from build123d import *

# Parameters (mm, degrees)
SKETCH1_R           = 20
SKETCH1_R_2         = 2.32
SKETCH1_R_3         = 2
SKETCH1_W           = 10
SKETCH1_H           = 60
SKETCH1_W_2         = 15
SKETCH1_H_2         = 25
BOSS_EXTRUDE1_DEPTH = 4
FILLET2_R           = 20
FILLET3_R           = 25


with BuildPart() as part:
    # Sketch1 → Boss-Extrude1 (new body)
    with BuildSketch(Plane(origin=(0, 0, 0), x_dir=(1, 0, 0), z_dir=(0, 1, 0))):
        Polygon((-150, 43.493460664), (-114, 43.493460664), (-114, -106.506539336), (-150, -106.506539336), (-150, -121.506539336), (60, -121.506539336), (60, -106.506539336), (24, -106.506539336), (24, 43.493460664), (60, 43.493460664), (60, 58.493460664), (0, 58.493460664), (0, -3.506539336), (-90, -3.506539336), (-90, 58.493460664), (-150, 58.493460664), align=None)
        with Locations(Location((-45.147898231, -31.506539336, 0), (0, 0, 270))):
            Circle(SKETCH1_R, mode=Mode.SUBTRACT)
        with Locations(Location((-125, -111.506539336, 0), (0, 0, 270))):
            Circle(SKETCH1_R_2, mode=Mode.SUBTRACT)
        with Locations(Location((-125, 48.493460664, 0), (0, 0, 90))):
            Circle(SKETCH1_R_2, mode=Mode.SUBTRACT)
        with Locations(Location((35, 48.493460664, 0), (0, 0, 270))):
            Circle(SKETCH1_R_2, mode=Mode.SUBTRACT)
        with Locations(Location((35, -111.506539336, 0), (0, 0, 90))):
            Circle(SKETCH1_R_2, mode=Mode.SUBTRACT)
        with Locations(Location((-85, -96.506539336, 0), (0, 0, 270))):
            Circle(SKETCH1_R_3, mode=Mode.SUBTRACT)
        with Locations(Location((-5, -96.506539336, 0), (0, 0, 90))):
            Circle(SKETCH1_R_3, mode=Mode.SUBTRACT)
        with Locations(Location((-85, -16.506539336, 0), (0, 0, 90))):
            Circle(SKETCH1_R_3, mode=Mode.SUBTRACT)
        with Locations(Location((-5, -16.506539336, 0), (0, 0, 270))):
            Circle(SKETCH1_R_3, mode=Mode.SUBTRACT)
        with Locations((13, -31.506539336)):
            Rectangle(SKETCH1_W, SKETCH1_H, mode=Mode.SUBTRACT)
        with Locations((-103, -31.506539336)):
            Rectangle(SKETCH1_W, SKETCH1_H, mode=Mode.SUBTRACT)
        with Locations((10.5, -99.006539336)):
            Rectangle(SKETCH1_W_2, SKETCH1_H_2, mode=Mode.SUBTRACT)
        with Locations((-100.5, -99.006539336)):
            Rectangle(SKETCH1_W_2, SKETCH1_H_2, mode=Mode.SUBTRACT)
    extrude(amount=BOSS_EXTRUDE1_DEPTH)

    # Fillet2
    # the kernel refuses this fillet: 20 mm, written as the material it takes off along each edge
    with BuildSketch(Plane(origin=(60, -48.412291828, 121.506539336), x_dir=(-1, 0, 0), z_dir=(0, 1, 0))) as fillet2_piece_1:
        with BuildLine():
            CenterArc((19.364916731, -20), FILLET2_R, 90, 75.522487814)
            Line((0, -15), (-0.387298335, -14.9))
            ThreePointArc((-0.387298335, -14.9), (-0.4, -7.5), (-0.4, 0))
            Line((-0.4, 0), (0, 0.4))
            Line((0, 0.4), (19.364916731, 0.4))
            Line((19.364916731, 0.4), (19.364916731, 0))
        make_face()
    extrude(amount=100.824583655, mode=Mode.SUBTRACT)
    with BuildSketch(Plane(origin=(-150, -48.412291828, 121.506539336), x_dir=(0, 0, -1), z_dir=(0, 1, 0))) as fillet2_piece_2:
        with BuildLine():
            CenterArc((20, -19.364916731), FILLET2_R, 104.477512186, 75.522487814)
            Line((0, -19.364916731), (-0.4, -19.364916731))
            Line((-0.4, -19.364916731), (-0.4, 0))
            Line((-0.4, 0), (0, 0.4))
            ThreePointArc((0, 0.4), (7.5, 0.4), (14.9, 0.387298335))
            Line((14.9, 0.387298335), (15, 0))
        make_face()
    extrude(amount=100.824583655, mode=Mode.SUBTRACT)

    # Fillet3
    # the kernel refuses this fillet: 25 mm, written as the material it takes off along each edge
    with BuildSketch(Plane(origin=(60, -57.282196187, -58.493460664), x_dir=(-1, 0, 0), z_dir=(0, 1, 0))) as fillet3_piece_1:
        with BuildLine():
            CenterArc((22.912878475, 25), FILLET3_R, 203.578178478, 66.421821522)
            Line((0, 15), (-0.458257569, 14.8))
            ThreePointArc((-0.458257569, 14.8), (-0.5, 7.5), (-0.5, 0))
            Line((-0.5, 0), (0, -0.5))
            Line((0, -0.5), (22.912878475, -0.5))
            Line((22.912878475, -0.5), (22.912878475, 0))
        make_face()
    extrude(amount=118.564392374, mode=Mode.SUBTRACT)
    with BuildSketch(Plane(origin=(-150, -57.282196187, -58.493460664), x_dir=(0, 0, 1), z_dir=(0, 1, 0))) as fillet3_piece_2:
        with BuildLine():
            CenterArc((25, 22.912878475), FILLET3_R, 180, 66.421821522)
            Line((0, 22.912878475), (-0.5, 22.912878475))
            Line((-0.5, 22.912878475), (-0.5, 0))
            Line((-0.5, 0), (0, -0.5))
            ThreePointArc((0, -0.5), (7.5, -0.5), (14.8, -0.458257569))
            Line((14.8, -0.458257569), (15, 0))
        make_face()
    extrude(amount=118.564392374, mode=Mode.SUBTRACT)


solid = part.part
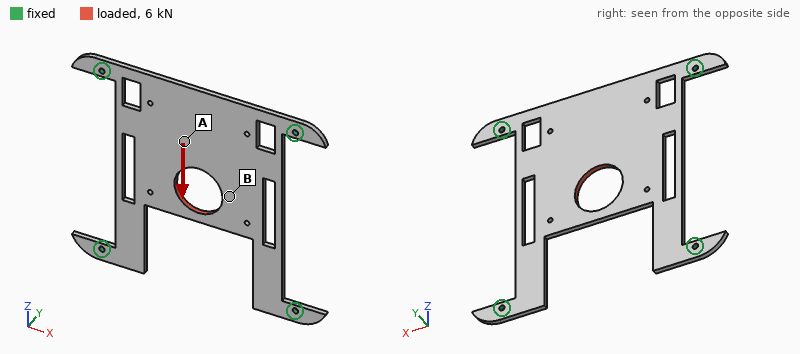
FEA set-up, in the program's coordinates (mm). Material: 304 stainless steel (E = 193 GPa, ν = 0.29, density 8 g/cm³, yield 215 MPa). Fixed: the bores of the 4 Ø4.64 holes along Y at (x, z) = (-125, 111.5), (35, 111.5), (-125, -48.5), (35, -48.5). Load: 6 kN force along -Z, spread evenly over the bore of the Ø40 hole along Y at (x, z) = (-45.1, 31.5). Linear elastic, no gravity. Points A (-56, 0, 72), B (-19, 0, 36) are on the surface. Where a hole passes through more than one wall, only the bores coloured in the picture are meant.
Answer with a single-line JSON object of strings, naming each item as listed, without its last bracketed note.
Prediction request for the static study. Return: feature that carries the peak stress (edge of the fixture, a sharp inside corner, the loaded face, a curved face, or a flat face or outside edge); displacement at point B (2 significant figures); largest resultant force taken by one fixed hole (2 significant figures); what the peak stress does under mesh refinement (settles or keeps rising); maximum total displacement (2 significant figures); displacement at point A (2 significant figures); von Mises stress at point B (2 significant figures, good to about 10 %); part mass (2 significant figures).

{"feature that carries the peak stress": "edge of the fixture", "displacement at point B": "30 µm", "largest resultant force taken by one fixed hole": "1.8 kN", "what the peak stress does under mesh refinement": "keeps rising", "maximum total displacement": "41 µm", "displacement at point A": "30 µm", "von Mises stress at point B": "30 MPa", "part mass": "570 g"}
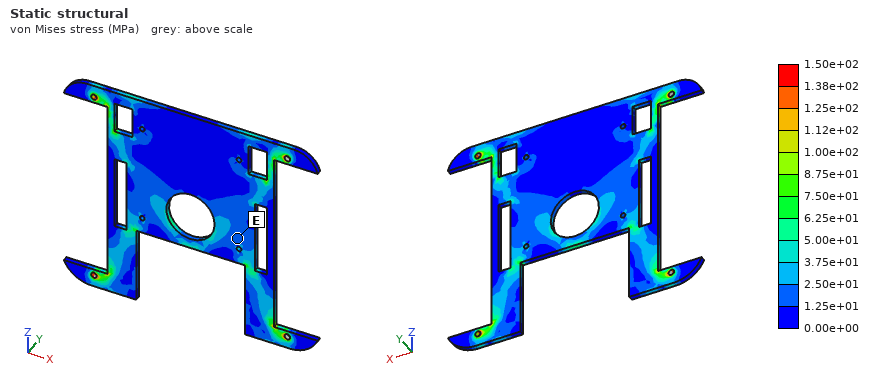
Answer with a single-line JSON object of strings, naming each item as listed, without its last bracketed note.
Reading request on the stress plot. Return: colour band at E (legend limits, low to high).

{"colour band at E": "1.25e+01 to 2.50e+01 MPa"}
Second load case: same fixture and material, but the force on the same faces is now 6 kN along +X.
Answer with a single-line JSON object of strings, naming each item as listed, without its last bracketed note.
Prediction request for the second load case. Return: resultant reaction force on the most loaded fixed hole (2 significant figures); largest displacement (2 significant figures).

{"resultant reaction force on the most loaded fixed hole": "2.8 kN", "largest displacement": "99 µm"}
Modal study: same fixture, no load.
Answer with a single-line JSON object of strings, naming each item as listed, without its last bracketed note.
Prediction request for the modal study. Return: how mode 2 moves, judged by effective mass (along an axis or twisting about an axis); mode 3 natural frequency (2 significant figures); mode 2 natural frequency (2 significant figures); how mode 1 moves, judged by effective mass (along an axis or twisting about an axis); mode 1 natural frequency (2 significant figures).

{"how mode 2 moves, judged by effective mass": "twisting about Z", "mode 3 natural frequency": "780 Hz", "mode 2 natural frequency": "720 Hz", "how mode 1 moves, judged by effective mass": "along Y", "mode 1 natural frequency": "380 Hz"}
